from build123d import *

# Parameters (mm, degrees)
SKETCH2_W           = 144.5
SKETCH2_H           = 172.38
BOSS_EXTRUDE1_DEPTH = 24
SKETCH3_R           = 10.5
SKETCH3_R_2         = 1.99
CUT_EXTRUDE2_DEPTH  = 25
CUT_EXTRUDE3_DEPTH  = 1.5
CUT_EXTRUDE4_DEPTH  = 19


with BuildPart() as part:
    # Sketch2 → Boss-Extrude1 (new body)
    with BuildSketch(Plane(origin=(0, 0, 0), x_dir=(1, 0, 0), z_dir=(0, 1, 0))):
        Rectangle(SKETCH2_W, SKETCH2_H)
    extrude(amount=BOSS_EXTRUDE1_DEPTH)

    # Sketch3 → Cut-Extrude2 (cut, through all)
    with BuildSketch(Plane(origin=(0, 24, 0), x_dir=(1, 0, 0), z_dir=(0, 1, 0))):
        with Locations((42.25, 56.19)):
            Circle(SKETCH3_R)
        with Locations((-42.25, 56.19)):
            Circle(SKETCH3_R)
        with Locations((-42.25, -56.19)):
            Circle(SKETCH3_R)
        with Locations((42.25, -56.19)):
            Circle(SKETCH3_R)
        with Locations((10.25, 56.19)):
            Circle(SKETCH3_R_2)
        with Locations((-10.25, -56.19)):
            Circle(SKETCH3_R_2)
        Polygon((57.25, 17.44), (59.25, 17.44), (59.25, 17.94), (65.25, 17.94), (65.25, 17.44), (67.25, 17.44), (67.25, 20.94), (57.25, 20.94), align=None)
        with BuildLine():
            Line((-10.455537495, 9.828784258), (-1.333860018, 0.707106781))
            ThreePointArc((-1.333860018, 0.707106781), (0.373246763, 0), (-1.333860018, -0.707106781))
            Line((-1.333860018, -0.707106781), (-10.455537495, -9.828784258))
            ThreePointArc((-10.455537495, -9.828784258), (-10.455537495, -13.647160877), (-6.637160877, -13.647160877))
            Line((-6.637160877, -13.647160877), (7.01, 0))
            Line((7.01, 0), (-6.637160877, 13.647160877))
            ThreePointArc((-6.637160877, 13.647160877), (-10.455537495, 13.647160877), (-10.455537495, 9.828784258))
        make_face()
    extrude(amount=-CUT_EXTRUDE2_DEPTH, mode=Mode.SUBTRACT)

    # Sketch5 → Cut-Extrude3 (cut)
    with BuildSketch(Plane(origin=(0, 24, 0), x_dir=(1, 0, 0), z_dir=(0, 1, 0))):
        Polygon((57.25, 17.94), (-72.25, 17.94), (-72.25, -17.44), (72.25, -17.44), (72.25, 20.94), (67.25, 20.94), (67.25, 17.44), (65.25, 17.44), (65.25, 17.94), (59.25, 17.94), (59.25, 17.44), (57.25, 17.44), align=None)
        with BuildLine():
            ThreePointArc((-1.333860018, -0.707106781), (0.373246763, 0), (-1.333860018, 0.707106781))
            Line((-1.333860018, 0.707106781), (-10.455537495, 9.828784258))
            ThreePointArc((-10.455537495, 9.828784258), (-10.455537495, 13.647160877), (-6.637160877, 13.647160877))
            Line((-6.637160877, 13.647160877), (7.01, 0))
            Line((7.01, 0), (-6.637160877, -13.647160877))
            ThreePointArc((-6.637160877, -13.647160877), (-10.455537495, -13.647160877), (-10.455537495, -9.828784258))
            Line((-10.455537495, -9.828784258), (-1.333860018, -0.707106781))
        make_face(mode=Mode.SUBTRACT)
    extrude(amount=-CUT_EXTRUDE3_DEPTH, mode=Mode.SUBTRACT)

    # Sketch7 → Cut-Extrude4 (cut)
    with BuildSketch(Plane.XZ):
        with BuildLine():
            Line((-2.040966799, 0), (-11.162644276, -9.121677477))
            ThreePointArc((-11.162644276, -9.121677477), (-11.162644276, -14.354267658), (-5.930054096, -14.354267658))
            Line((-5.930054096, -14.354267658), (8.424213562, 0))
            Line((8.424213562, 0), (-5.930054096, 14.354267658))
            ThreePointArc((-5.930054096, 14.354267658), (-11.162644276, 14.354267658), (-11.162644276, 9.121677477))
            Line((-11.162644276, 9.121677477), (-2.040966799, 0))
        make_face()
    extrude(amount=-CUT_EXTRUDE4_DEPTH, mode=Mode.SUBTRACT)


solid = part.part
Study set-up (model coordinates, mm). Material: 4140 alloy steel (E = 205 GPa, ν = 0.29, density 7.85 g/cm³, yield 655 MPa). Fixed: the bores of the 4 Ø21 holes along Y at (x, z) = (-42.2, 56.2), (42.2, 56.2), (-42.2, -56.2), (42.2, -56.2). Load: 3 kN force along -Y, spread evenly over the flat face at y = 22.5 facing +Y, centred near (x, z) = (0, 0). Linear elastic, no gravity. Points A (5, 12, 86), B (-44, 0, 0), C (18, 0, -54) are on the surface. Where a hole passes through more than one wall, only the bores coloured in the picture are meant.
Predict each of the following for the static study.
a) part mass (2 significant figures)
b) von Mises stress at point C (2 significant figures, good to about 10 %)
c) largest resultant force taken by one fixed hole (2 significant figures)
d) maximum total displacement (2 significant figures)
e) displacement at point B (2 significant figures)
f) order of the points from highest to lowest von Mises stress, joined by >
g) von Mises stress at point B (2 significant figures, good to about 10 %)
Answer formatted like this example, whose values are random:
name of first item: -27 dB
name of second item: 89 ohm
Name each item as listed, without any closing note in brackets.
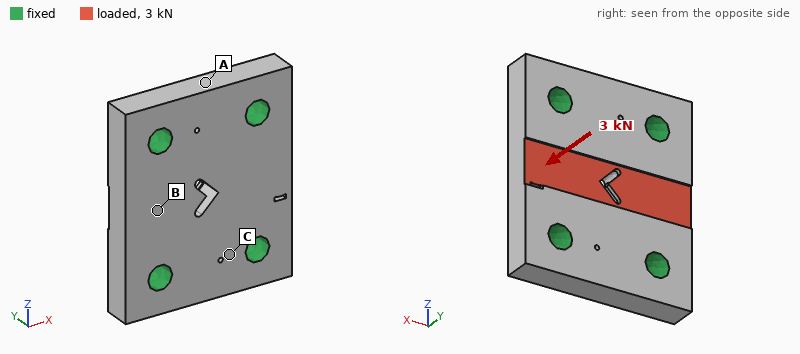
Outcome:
part mass: 4.3 kg
von Mises stress at point C: 0.98 MPa
largest resultant force taken by one fixed hole: 760 N
maximum total displacement: 1.3 µm
displacement at point B: 0.81 µm
order of the points from highest to lowest von Mises stress, joined by >: B > C > A
von Mises stress at point B: 2.3 MPa
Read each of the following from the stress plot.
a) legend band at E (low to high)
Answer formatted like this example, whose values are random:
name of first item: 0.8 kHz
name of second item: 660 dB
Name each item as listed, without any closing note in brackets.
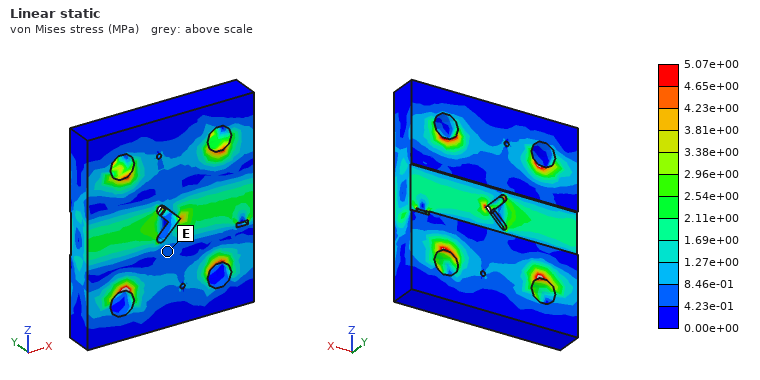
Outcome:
legend band at E: 4.23e-01 to 8.46e-01 MPa
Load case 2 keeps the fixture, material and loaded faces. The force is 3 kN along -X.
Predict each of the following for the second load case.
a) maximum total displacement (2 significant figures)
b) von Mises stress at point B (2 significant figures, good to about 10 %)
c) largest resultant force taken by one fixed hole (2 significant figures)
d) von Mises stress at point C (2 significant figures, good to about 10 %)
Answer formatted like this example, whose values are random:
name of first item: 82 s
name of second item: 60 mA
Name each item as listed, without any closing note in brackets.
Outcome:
maximum total displacement: 0.71 µm
von Mises stress at point B: 0.33 MPa
largest resultant force taken by one fixed hole: 820 N
von Mises stress at point C: 0.48 MPa
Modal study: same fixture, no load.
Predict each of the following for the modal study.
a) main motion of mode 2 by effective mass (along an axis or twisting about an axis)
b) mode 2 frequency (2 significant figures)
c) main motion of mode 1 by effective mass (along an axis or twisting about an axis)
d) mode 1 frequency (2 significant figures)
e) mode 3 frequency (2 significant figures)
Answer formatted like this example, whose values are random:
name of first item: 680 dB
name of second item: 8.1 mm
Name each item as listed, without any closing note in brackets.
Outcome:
main motion of mode 2 by effective mass: twisting about Z
mode 2 frequency: 9400 Hz
main motion of mode 1 by effective mass: along Y
mode 1 frequency: 8200 Hz
mode 3 frequency: 11 kHz
